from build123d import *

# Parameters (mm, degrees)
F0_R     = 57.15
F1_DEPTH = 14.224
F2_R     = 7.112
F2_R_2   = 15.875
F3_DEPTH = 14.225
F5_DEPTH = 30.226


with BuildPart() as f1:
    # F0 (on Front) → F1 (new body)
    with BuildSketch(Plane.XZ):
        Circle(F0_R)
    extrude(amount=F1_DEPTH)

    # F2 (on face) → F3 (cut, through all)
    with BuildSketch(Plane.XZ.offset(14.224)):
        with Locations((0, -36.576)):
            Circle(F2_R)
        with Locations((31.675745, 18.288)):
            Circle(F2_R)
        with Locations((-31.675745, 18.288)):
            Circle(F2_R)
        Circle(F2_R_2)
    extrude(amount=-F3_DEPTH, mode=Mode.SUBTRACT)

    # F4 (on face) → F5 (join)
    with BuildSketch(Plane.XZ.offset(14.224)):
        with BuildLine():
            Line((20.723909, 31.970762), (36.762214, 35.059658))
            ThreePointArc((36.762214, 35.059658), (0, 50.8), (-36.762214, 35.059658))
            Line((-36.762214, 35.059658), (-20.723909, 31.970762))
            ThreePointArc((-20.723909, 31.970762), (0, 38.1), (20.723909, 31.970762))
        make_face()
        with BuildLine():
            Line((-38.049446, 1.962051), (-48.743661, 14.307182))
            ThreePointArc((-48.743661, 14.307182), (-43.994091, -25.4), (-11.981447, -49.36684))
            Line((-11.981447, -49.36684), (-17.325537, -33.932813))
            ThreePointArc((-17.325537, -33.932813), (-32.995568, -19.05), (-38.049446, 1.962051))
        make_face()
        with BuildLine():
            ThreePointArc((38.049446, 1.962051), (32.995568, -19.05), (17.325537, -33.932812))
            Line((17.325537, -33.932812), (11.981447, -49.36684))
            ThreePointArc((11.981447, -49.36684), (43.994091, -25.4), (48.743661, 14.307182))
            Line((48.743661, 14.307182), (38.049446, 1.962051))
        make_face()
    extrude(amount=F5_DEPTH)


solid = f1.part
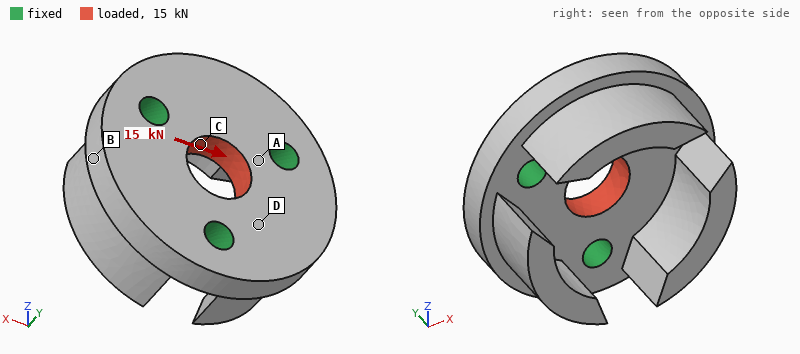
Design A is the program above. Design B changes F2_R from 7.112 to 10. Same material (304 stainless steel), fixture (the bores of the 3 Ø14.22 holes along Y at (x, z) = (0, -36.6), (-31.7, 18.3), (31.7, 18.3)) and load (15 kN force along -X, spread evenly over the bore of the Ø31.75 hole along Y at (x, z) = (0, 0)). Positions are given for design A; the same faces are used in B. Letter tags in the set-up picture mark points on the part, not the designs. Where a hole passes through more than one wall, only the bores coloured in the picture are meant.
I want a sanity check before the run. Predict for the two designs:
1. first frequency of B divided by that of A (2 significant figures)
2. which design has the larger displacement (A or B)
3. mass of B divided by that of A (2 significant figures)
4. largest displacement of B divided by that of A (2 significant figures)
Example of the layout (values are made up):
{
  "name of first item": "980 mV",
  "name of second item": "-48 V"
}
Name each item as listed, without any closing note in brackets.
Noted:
{
  "first frequency of B divided by that of A": "1.1",
  "which design has the larger displacement": "A",
  "mass of B divided by that of A": "0.97",
  "largest displacement of B divided by that of A": "0.84"
}
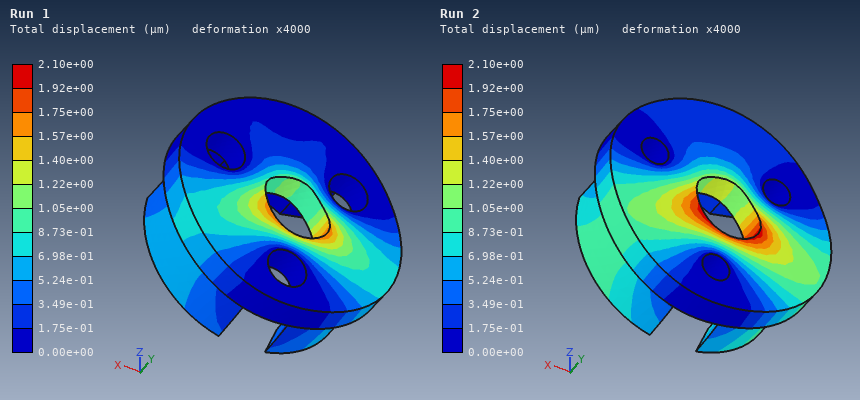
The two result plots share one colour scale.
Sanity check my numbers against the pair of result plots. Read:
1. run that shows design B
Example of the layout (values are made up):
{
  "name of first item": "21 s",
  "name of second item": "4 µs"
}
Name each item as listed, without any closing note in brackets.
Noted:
{
  "run that shows design B": "Run 1"
}
